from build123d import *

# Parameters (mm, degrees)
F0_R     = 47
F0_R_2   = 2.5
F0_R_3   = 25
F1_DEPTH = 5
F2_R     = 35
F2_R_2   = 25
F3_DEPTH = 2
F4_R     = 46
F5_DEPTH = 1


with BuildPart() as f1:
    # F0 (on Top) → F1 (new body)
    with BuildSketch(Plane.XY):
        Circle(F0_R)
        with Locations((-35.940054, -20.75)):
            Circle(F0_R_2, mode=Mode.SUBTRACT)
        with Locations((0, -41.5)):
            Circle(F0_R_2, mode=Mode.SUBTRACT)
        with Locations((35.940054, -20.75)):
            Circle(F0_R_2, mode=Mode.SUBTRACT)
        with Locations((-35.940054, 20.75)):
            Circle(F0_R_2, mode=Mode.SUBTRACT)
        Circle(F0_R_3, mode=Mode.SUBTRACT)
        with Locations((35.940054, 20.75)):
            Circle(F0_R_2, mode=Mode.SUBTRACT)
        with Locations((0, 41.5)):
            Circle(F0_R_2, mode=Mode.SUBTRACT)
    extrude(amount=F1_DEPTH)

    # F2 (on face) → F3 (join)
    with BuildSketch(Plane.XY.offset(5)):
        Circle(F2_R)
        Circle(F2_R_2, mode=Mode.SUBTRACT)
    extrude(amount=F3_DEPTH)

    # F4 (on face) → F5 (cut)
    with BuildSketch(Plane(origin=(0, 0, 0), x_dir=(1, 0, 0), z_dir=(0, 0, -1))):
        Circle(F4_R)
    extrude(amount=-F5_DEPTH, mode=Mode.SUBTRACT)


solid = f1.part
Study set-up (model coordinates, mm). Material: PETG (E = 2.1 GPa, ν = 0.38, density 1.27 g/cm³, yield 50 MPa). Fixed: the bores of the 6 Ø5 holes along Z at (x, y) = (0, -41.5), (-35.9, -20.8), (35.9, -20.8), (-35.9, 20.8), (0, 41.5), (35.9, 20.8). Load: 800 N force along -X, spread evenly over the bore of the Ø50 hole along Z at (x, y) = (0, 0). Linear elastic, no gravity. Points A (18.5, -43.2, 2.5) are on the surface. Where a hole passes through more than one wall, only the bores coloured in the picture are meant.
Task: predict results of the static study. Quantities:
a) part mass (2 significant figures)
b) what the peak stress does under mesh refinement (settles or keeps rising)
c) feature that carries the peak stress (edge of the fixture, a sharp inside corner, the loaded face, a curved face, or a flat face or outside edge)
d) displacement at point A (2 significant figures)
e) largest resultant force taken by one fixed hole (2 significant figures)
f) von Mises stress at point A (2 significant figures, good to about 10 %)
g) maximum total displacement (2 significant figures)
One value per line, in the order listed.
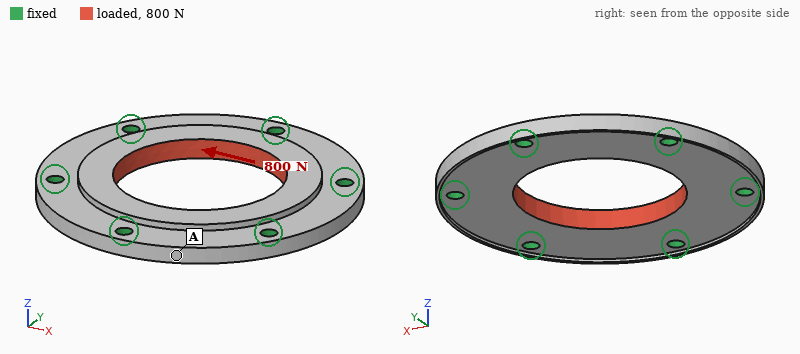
30 g
keeps rising
edge of the fixture
8.0 µm
150 N
0.67 MPa
38 µm
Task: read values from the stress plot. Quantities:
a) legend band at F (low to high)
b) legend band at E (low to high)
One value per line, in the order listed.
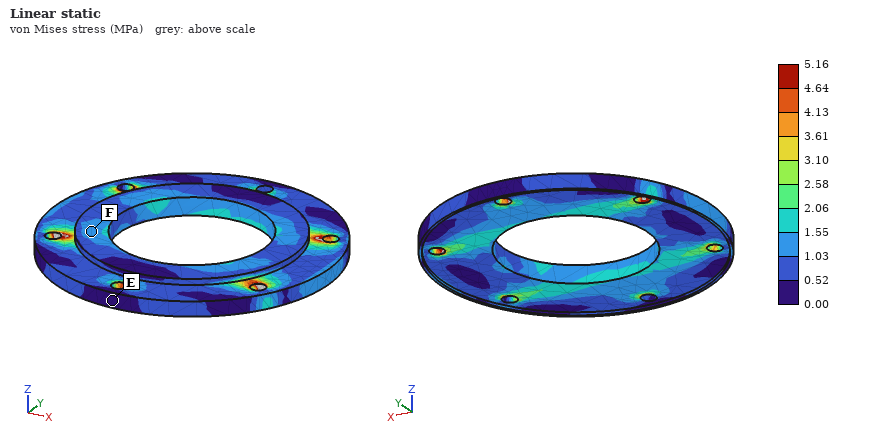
1.03 to 1.55 MPa
0.00 to 0.52 MPa
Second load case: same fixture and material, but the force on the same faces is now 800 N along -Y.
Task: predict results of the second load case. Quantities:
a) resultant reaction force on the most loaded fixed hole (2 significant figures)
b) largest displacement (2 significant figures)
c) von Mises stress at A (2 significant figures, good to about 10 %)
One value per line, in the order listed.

170 N
34 µm
0.98 MPa
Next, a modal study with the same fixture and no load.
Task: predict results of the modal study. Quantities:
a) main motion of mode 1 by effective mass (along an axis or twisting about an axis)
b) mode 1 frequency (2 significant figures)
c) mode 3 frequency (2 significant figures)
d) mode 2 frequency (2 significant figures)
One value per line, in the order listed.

along Z
2500 Hz
3000 Hz
3000 Hz
